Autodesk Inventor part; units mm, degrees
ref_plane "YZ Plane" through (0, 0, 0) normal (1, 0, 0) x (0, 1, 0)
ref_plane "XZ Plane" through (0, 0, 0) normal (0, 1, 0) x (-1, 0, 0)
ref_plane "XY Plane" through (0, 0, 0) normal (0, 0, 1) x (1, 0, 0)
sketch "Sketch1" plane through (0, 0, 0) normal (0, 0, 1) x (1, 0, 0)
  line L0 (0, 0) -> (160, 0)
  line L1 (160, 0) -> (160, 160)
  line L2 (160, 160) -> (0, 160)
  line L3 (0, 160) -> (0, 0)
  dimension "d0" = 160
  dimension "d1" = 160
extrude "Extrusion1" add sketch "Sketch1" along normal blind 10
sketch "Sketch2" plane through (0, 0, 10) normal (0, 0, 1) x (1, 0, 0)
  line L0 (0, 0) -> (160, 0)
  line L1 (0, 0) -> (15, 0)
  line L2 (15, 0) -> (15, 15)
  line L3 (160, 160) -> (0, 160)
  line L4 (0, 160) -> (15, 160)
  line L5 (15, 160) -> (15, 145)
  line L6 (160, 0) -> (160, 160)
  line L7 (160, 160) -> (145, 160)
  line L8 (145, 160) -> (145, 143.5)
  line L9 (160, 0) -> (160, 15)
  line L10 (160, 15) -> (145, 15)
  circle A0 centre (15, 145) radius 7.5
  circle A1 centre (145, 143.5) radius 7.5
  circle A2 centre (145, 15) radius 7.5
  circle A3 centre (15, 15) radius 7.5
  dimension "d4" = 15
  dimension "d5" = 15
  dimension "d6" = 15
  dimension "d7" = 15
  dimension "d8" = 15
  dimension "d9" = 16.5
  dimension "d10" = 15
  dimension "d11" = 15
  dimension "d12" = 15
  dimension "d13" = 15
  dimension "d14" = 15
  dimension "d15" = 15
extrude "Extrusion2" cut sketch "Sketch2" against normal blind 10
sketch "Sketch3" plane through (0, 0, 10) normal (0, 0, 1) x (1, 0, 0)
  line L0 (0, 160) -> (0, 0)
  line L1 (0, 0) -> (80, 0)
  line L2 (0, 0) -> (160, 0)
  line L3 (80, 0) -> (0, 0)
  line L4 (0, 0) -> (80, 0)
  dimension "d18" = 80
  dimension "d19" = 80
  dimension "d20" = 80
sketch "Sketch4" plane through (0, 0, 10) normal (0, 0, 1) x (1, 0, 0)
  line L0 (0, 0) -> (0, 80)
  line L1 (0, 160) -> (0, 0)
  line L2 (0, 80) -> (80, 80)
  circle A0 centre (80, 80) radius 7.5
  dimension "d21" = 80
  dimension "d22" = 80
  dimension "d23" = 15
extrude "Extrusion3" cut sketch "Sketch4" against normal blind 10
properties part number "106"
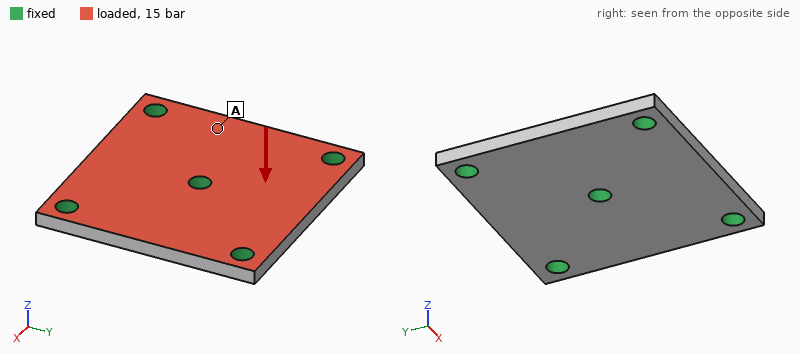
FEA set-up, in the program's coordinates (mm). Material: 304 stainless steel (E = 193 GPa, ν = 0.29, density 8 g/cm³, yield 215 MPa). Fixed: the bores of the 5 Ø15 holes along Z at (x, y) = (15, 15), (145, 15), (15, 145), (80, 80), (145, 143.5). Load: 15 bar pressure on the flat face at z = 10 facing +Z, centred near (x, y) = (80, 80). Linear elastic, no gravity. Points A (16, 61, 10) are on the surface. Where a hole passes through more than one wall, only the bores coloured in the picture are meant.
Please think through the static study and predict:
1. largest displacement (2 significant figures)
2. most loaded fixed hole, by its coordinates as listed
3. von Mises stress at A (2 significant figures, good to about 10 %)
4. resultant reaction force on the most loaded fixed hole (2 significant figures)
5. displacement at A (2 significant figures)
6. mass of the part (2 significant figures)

44 µm
(80, 80)
29 MPa
13 kN
31 µm
2.0 kg
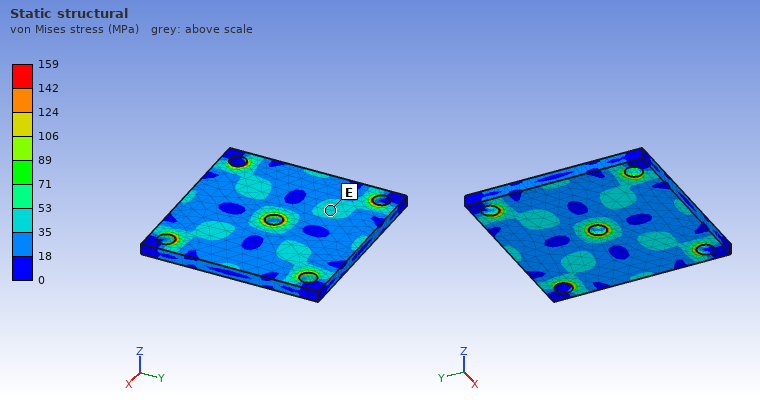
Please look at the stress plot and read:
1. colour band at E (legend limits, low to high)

35 to 53 MPa
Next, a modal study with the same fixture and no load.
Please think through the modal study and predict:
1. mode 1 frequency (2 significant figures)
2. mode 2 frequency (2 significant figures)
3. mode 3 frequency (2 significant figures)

3800 Hz
4000 Hz
4000 Hz
